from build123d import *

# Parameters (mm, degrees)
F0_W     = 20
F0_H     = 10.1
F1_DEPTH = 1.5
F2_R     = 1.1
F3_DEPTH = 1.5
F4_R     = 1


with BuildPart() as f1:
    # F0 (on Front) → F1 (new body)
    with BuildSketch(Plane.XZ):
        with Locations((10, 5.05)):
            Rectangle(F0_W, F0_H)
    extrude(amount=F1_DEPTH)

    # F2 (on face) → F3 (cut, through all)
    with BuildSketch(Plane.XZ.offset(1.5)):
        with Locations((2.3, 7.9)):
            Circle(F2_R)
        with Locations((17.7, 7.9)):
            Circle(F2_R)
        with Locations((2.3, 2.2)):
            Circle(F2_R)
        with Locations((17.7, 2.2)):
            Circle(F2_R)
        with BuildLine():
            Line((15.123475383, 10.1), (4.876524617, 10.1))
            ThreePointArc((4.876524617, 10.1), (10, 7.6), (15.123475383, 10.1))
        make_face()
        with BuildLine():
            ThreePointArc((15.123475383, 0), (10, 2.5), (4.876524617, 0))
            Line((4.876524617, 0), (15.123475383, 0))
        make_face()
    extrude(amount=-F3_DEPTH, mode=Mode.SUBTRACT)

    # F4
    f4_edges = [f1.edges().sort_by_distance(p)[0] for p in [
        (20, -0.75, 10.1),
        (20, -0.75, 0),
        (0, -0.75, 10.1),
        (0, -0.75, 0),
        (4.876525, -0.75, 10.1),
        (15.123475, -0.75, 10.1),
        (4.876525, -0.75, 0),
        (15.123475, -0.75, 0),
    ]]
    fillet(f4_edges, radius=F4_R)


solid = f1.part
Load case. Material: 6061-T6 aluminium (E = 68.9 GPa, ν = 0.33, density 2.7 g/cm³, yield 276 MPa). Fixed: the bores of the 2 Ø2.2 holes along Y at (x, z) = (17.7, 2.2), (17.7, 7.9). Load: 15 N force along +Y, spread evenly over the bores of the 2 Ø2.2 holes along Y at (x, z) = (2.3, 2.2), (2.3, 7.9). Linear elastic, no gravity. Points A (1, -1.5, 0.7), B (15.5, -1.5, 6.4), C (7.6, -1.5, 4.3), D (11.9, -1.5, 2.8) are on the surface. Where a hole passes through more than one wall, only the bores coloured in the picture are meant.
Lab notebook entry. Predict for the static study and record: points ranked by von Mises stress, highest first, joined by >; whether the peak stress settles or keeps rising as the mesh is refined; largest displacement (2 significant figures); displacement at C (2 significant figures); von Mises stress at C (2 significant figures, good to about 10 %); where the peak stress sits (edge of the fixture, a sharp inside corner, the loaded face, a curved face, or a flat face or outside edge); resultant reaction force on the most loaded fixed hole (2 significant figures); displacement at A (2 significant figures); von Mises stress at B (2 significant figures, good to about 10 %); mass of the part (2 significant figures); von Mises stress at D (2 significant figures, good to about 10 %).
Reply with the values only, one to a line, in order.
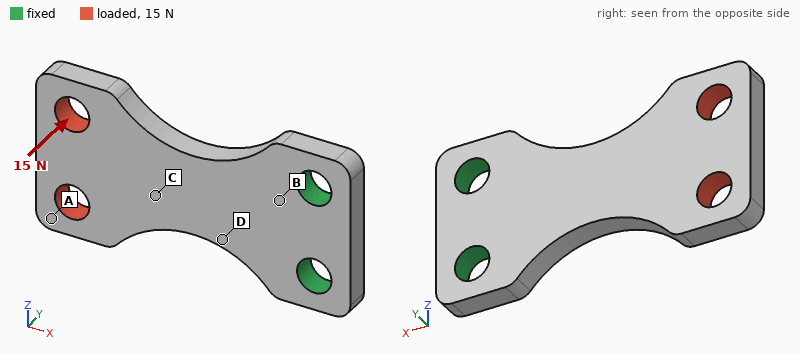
D > B > C > A
keeps rising
0.15 mm
0.055 mm
35 MPa
edge of the fixture
7.5 N
0.13 mm
54 MPa
0.61 g
72 MPa
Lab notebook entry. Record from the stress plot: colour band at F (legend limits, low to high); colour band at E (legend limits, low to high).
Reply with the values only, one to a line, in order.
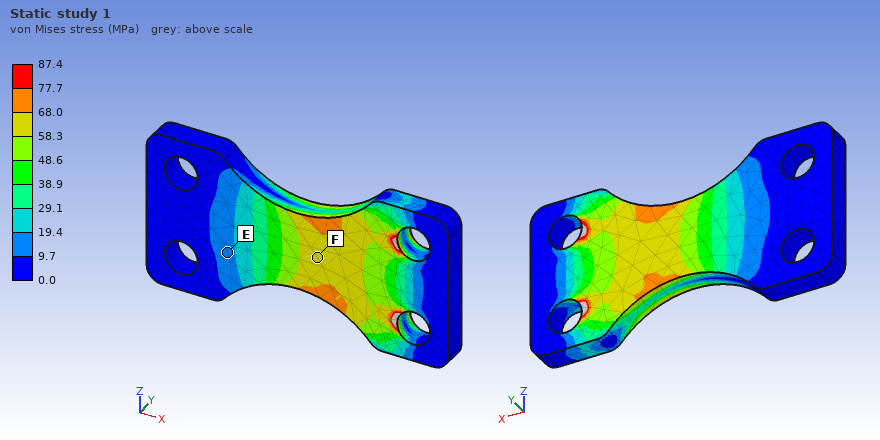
58.3 to 68.0 MPa
9.7 to 19.4 MPa
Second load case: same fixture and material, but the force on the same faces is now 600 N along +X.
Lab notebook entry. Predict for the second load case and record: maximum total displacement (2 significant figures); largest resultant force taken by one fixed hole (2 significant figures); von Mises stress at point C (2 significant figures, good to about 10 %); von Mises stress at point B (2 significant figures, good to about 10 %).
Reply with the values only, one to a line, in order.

16 µm
310 N
58 MPa
54 MPa
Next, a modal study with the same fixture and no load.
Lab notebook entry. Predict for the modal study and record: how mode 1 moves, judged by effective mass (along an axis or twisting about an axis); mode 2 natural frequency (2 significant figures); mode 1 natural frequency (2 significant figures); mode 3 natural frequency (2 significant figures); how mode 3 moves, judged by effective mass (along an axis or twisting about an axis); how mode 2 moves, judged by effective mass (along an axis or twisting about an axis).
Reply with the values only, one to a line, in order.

along Y
14 kHz
4000 Hz
15 kHz
along Z
twisting about X
